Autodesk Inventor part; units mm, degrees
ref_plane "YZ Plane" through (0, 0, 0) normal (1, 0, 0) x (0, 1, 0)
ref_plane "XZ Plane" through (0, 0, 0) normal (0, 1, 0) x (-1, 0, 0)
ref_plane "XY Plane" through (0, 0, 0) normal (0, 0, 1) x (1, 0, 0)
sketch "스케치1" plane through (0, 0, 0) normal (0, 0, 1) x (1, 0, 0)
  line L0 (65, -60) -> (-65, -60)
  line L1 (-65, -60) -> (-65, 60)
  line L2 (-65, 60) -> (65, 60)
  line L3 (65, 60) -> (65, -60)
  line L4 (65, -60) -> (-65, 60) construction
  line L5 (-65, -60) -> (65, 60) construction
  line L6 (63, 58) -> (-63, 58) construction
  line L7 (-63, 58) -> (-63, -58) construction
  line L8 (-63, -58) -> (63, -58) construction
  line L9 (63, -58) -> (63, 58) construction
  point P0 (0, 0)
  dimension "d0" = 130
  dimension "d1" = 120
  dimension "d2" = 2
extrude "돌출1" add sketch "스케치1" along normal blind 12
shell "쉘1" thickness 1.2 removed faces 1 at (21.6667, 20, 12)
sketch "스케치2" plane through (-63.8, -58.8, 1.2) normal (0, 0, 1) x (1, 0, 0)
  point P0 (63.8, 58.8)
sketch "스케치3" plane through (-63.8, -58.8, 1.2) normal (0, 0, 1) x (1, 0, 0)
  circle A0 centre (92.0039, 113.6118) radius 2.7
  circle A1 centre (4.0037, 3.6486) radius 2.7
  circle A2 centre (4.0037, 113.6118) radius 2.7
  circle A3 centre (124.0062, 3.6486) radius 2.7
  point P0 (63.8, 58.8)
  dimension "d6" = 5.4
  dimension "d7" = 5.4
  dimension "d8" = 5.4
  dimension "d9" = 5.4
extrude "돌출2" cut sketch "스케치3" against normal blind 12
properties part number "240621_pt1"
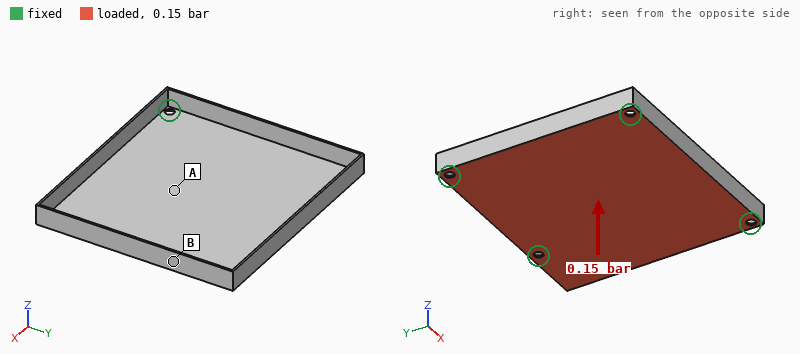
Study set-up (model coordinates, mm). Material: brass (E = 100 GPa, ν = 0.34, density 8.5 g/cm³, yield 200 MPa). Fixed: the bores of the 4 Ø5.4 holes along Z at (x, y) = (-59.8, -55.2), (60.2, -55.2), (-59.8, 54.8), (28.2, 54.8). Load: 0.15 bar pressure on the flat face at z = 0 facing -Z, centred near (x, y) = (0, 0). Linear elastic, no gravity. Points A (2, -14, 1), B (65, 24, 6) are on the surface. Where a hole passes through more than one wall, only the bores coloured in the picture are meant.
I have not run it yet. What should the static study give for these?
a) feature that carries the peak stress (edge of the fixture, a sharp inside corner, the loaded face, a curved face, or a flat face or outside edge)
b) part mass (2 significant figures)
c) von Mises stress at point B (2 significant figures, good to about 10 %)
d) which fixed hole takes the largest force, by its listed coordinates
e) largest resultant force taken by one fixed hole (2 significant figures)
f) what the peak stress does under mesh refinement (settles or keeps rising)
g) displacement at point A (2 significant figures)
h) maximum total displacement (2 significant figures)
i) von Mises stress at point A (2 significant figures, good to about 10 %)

edge of the fixture
210 g
16 MPa
(28.2, 54.8)
84 N
keeps rising
0.52 mm
0.54 mm
32 MPa
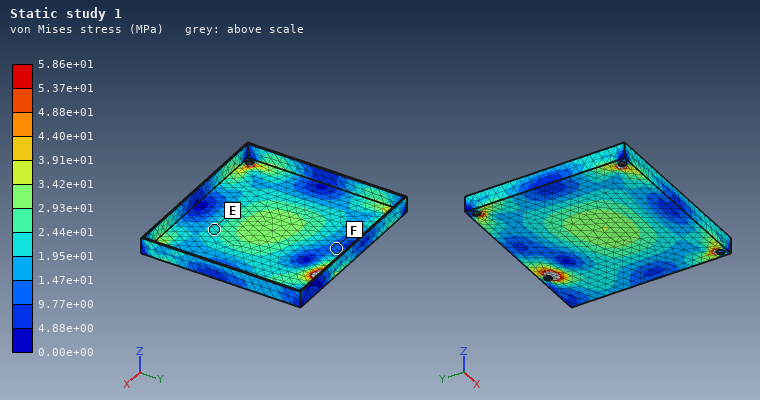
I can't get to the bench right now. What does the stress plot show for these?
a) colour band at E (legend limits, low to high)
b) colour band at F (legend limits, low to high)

1.95e+01 to 2.44e+01 MPa
9.77e+00 to 1.47e+01 MPa
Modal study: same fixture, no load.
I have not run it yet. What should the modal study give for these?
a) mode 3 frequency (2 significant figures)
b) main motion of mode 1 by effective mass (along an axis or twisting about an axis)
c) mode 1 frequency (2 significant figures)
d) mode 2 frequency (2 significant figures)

780 Hz
along Z
330 Hz
670 Hz
